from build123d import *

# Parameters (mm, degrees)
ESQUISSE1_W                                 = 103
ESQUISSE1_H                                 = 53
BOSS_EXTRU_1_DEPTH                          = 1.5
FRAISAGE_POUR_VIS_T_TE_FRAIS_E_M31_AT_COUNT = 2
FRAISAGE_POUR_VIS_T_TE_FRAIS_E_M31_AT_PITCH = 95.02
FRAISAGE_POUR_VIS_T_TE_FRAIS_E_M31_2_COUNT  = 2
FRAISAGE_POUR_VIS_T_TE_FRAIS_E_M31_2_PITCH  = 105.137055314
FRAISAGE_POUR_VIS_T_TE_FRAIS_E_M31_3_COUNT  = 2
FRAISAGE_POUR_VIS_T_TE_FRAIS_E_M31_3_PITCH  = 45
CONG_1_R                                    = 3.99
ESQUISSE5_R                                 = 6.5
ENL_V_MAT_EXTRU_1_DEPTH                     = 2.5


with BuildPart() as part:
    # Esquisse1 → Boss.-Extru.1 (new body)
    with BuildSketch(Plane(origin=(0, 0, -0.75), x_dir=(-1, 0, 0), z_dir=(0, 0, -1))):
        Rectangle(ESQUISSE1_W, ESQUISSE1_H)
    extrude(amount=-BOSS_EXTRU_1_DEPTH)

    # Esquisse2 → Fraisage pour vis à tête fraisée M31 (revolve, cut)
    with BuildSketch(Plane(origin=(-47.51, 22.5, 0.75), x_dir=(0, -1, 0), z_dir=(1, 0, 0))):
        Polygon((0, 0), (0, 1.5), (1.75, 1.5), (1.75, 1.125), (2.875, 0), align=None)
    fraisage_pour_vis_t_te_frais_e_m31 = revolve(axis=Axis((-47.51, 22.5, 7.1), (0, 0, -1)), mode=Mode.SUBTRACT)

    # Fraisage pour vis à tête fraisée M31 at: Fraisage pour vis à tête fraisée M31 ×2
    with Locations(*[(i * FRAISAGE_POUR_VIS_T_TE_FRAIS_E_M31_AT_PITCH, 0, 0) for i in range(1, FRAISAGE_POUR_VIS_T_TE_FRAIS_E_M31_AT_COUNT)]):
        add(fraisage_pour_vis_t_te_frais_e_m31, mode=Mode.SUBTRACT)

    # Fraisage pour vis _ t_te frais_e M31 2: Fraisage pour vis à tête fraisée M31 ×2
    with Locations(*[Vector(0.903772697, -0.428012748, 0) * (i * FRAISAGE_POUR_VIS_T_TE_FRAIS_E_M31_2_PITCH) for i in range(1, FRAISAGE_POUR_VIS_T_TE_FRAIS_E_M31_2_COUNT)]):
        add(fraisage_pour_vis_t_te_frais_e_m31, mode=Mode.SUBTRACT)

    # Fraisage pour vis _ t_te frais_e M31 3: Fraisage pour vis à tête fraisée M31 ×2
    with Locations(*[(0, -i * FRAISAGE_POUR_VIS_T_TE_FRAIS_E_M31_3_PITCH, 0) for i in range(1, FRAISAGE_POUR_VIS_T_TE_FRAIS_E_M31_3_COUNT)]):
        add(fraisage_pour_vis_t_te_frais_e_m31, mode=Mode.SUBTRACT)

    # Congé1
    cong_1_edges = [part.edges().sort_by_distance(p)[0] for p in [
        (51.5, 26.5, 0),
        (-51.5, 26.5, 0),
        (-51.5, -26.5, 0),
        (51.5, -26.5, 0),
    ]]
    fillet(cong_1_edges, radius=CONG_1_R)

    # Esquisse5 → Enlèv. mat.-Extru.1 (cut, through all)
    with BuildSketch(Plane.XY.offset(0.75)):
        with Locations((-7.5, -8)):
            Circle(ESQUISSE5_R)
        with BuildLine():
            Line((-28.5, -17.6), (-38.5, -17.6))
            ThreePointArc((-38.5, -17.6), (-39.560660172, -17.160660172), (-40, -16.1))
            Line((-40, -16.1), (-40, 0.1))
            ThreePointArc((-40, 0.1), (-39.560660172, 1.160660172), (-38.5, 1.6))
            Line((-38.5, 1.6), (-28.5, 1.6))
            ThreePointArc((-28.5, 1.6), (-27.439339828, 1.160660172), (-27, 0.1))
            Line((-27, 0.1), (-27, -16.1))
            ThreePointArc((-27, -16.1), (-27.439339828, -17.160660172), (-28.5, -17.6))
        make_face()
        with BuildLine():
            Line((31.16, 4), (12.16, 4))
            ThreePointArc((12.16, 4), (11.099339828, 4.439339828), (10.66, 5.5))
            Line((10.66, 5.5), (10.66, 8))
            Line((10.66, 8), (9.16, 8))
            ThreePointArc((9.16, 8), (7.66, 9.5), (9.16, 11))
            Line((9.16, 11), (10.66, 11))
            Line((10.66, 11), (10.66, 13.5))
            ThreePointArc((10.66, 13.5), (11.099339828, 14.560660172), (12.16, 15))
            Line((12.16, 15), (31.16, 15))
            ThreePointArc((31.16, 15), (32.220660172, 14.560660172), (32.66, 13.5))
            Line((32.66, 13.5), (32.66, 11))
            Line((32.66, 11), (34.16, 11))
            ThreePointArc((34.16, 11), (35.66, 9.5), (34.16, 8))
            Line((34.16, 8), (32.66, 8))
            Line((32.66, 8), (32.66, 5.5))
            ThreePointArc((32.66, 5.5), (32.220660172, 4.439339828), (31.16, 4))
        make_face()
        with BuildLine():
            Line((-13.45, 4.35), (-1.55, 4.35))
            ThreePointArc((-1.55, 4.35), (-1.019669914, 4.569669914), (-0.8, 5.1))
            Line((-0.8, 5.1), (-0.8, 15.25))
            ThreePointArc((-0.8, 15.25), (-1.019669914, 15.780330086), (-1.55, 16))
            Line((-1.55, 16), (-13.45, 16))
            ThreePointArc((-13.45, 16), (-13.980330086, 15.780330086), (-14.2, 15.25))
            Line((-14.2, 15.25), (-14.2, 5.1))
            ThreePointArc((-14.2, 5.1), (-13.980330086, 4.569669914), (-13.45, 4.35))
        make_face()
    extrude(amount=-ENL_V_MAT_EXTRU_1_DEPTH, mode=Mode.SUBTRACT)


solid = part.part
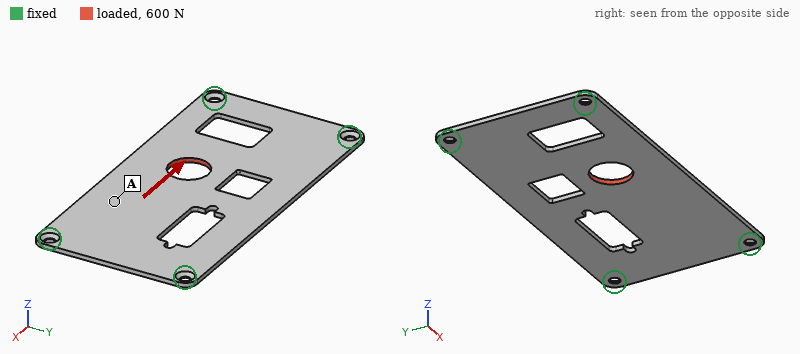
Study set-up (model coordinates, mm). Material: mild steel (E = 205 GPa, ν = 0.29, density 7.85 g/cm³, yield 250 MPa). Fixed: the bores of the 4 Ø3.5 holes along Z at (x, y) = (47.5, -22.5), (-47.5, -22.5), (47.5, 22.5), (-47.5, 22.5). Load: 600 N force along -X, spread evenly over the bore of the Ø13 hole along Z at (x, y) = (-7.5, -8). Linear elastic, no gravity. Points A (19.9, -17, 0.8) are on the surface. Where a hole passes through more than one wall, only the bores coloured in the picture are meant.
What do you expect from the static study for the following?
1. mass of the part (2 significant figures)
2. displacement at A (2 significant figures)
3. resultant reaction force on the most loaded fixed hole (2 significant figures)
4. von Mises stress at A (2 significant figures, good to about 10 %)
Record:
54 g
3.2 µm
190 N
4.9 MPa
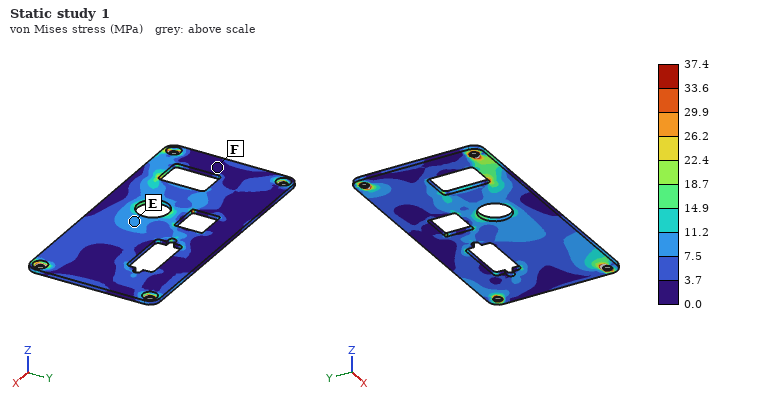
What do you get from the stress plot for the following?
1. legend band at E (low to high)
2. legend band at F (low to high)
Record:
7.5 to 11.2 MPa
0.0 to 3.7 MPa
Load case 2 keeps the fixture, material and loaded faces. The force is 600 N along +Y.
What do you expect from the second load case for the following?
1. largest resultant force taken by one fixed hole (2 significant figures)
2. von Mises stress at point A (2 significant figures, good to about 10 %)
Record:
240 N
7.7 MPa
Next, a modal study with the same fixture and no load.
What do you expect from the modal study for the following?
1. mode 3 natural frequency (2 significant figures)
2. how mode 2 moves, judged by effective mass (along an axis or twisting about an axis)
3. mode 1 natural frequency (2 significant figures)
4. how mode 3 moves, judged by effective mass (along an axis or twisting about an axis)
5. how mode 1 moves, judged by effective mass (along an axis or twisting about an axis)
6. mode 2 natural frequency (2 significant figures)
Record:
1900 Hz
twisting about X
690 Hz
twisting about Y
along Z
1200 Hz
